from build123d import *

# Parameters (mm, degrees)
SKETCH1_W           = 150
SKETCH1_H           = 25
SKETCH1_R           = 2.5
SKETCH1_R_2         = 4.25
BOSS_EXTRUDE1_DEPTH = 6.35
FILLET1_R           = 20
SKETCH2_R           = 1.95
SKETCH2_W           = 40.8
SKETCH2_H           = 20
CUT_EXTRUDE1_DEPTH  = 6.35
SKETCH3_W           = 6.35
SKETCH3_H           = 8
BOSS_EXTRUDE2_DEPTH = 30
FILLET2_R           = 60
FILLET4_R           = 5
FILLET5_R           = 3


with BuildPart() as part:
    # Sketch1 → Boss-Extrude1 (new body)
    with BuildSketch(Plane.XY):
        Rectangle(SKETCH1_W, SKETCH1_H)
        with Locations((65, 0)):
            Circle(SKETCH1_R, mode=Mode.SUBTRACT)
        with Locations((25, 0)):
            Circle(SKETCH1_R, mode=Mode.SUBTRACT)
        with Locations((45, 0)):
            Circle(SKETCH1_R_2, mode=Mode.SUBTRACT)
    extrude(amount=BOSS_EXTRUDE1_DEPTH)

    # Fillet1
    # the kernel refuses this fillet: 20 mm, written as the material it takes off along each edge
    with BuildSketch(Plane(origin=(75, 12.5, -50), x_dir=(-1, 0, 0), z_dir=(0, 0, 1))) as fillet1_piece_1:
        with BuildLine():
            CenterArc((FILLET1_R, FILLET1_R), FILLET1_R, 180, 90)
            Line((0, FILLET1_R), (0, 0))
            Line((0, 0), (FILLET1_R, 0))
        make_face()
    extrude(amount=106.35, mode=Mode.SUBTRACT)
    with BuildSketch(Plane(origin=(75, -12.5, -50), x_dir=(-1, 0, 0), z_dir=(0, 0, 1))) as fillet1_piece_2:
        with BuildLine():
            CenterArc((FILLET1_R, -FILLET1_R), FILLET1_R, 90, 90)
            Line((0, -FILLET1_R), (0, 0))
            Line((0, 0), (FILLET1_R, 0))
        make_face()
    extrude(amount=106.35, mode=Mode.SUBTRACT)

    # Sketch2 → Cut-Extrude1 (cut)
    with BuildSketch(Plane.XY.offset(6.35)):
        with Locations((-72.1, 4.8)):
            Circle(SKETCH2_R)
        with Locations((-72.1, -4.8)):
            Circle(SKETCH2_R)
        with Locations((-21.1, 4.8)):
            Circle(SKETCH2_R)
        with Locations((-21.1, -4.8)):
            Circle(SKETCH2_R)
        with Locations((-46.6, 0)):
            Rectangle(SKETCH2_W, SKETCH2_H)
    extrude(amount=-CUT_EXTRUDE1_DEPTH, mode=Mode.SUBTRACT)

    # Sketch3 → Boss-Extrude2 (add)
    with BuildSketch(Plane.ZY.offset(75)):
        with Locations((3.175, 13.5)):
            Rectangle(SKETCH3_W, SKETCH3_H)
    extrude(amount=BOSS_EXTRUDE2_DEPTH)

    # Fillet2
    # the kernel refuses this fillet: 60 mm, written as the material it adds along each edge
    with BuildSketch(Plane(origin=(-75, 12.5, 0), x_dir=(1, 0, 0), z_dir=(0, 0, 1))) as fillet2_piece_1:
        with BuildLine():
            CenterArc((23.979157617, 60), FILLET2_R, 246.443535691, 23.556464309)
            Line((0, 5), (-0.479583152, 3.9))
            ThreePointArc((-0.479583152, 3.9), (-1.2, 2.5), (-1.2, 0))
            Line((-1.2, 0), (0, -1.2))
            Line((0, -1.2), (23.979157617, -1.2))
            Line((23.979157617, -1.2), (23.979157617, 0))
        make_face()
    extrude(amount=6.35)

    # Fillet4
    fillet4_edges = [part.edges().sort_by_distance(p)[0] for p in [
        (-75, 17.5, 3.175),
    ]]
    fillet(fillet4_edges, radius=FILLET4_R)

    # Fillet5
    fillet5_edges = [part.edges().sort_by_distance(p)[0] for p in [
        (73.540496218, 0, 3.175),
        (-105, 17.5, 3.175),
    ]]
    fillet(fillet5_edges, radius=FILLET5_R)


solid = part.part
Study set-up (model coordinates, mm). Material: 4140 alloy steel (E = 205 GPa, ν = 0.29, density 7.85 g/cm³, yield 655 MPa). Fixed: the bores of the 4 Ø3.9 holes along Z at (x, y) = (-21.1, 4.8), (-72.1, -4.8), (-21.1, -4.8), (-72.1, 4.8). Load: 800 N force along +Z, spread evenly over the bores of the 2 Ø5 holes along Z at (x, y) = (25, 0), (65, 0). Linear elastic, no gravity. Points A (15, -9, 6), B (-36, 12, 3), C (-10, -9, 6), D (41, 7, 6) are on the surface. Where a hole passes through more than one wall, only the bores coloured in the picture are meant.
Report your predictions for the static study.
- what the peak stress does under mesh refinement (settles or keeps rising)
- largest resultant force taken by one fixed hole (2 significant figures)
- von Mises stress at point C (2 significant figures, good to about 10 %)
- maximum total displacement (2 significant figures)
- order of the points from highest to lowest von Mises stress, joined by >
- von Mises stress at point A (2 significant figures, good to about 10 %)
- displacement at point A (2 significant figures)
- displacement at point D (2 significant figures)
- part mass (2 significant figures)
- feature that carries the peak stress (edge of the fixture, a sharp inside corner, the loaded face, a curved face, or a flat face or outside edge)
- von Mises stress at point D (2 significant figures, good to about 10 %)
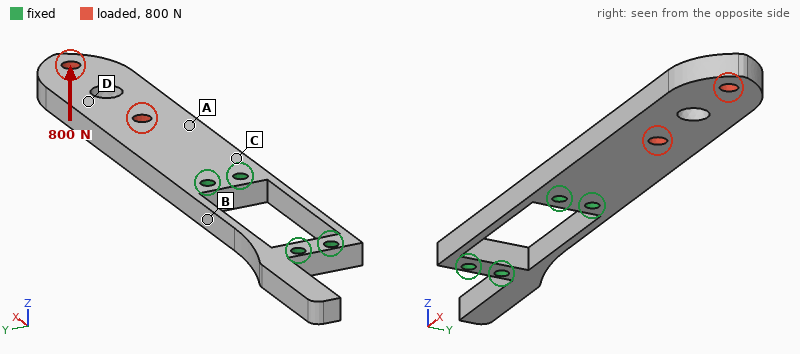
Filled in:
keeps rising
420 N
260 MPa
1.2 mm
C > A > D > B
150 MPa
0.25 mm
0.64 mm
140 g
edge of the fixture
77 MPa
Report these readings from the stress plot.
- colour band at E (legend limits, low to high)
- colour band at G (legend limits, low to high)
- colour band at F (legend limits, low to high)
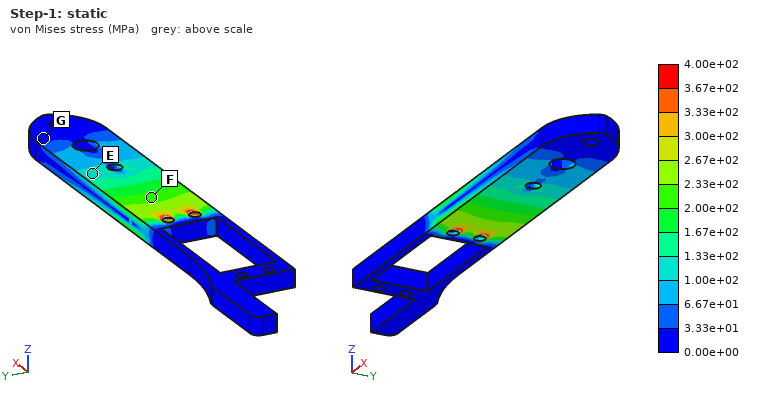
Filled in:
1.00e+02 to 1.33e+02 MPa
0.00e+00 to 3.33e+01 MPa
2.00e+02 to 2.33e+02 MPa
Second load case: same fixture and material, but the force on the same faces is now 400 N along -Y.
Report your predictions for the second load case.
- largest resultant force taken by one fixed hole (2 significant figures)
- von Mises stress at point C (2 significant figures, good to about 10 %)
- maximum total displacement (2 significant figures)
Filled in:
1.9 kN
25 MPa
50 µm
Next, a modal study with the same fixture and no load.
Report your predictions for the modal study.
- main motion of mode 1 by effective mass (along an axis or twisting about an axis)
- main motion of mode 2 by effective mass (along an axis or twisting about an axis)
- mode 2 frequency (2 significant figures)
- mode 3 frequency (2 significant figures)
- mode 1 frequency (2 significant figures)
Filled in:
along Z
along Y
2300 Hz
3600 Hz
680 Hz
